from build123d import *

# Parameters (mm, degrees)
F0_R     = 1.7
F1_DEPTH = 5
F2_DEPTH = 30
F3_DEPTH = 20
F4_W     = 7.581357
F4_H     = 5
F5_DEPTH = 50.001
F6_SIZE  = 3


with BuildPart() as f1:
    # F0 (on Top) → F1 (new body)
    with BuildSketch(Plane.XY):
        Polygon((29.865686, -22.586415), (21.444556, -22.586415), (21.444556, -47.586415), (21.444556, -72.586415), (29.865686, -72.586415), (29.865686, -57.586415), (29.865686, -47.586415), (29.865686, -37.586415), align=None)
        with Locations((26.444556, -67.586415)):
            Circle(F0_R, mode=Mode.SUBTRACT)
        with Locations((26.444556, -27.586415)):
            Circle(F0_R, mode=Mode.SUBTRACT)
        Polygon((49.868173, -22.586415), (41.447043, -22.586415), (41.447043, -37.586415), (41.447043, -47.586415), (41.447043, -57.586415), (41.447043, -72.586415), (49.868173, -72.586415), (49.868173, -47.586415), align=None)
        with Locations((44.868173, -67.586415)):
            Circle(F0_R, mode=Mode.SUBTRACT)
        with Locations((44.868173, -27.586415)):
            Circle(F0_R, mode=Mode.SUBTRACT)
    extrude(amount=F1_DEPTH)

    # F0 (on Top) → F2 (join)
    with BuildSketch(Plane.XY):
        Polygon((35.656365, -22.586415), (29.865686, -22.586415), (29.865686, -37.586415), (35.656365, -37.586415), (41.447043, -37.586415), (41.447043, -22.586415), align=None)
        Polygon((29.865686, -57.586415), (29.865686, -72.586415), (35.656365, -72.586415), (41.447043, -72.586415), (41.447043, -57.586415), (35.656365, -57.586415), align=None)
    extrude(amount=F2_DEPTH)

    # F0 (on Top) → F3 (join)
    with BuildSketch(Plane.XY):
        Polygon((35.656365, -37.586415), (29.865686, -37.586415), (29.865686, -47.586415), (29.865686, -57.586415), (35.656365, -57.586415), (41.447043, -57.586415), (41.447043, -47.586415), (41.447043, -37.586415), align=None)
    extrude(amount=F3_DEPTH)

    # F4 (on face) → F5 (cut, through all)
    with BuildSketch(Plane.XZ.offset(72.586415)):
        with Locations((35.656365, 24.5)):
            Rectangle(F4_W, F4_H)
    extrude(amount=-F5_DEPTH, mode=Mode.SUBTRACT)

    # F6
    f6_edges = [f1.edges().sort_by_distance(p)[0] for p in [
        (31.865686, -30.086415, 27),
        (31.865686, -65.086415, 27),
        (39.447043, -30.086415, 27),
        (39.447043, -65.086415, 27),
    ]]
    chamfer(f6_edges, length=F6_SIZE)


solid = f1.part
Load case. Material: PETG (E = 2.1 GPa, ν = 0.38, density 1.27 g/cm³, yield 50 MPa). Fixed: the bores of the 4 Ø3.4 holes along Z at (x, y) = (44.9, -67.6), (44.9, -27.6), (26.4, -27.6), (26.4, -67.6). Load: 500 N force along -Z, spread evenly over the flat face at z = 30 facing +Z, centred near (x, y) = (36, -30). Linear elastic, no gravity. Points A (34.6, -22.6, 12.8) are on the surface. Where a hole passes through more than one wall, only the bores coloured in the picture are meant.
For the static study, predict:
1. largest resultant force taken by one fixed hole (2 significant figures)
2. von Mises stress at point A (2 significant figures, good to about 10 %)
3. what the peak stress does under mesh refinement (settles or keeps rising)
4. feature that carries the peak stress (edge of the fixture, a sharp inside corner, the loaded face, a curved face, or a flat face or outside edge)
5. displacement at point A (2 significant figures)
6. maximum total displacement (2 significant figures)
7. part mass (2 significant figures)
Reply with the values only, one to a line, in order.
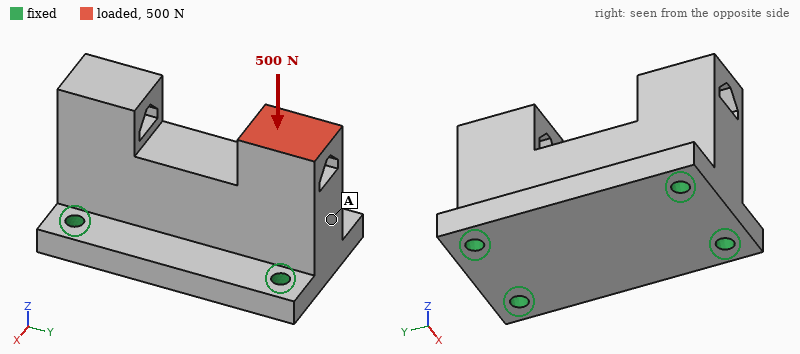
240 N
2.7 MPa
keeps rising
edge of the fixture
0.054 mm
0.12 mm
23 g
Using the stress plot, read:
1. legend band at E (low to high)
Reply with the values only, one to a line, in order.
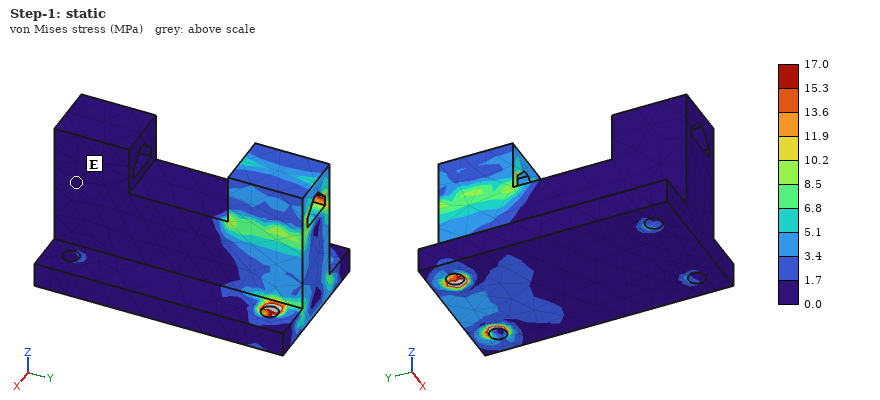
0.0 to 1.7 MPa
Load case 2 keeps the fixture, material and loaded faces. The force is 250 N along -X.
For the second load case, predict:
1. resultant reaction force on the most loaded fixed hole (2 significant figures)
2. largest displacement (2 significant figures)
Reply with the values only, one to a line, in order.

330 N
0.55 mm
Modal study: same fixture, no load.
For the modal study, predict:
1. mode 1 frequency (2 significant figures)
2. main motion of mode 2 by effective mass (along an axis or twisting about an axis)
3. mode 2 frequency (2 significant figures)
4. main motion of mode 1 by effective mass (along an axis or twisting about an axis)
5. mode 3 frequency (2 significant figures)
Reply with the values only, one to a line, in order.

2500 Hz
twisting about Z
3400 Hz
along X
4300 Hz
